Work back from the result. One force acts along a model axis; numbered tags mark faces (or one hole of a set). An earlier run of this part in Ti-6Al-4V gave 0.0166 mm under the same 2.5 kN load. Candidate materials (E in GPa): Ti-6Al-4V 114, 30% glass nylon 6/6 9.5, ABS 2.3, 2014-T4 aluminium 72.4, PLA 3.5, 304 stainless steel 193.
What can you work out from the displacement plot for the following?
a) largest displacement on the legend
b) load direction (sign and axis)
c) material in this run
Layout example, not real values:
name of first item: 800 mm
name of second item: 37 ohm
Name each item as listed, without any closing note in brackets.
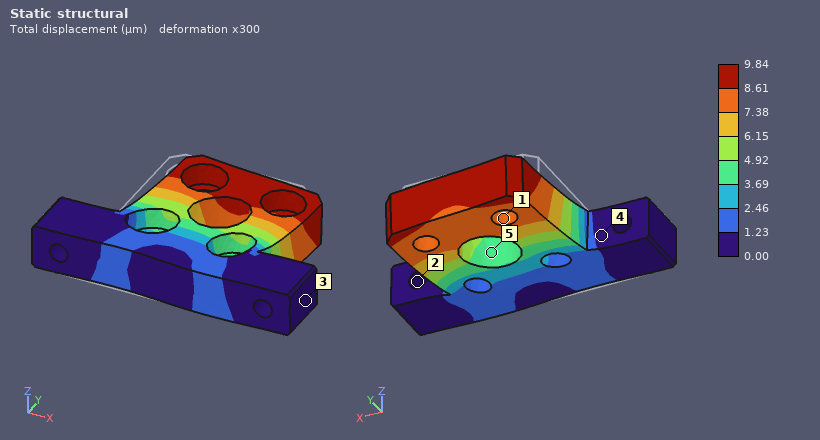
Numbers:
largest displacement on the legend: 9.84 µm
load direction: +X
material in this run: 304 stainless steel
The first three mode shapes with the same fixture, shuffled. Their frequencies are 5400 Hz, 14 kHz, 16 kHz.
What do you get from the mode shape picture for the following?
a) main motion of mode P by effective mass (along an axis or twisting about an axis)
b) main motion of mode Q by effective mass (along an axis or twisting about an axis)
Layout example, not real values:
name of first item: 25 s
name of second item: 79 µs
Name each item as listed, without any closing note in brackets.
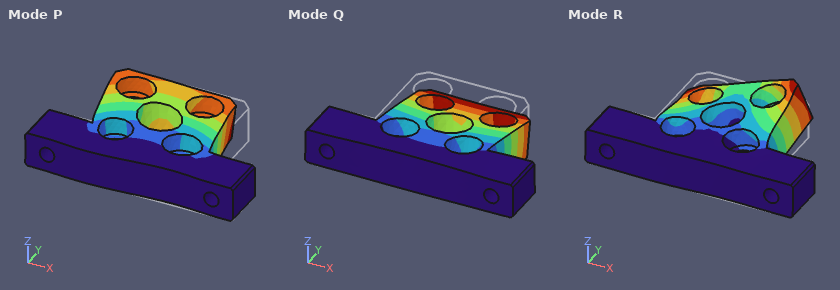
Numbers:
main motion of mode P by effective mass: along X
main motion of mode Q by effective mass: along Z
